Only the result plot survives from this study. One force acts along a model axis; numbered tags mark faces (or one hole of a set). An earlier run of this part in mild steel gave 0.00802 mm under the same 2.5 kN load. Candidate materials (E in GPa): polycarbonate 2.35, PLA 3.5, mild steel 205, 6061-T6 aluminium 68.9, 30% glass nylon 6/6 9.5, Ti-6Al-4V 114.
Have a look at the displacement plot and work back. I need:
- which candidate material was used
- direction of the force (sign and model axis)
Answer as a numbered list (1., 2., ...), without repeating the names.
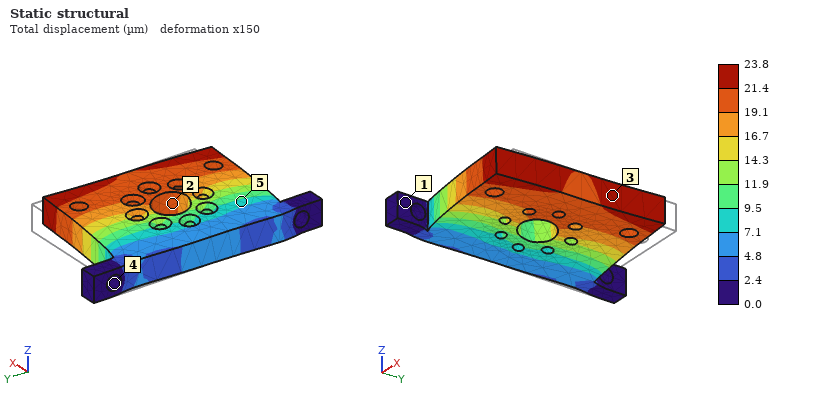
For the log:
1. 6061-T6 aluminium
2. -Y
